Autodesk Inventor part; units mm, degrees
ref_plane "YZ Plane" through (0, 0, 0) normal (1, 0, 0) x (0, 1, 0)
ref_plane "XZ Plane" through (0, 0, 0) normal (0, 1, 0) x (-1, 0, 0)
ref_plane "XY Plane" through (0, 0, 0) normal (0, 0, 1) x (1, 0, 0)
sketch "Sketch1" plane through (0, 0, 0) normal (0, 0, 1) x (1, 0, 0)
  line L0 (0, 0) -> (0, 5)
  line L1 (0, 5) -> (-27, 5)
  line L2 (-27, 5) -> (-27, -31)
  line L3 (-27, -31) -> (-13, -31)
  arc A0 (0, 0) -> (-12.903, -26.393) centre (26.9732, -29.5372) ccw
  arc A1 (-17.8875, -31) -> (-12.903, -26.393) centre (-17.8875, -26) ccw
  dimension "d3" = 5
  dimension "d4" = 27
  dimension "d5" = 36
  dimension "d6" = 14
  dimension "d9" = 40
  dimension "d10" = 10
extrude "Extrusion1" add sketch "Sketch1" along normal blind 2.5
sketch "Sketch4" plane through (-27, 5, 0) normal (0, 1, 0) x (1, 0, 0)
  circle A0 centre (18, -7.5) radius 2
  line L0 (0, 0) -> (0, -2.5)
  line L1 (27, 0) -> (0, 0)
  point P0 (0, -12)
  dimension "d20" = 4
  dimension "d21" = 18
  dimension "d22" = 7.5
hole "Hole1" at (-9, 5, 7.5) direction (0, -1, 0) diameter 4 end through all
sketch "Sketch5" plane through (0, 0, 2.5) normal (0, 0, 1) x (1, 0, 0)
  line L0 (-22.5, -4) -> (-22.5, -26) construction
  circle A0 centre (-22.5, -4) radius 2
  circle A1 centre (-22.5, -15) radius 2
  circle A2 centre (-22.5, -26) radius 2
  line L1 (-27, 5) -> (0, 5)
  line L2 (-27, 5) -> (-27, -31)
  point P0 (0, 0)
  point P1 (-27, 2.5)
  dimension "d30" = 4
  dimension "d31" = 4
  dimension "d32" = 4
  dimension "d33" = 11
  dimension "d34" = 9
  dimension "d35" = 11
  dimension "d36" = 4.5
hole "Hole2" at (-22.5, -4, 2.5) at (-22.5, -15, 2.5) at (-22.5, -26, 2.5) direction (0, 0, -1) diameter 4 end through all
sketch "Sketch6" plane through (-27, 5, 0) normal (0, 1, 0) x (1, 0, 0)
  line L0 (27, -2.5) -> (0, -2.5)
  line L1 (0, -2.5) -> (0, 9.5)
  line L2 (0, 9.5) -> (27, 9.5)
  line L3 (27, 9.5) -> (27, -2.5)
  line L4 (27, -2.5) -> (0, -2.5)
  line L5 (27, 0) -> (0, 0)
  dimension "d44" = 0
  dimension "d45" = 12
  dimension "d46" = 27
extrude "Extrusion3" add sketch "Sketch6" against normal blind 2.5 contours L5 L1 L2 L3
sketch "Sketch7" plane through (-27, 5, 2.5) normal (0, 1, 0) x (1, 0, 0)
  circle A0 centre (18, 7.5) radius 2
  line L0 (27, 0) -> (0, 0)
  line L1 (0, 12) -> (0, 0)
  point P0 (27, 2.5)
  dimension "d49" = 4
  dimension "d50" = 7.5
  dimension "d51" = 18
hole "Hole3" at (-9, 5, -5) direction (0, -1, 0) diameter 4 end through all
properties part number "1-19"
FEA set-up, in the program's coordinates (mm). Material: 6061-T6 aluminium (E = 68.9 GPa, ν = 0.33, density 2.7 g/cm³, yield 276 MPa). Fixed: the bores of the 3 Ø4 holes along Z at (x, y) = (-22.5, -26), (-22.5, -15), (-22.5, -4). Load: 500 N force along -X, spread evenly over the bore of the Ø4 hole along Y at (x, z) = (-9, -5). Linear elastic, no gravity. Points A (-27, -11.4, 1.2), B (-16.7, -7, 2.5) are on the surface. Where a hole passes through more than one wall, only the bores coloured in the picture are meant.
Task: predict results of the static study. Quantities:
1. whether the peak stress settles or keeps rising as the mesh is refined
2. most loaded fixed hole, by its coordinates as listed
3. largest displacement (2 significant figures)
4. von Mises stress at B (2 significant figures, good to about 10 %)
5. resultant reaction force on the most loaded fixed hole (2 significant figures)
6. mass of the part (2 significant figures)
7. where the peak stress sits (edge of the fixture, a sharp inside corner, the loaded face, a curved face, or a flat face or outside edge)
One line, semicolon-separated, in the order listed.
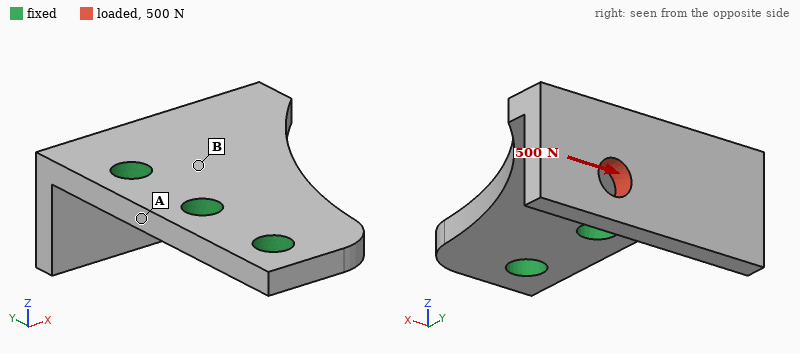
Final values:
keeps rising; (-22.5, -4); 0.20 mm; 66 MPa; 650 N; 6.0 g; edge of the fixture
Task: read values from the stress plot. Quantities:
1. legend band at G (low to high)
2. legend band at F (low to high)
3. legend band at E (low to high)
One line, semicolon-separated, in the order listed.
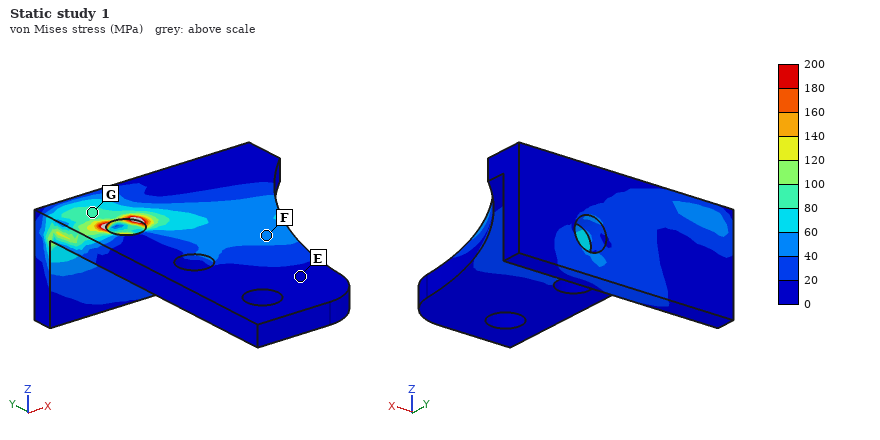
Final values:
80 to 100 MPa; 40 to 60 MPa; 0 to 20 MPa
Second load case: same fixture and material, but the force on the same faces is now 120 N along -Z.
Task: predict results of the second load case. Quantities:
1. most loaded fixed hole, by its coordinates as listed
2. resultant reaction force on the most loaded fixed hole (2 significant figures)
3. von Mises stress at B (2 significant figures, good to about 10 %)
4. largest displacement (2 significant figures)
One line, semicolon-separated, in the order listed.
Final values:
(-22.5, -4); 150 N; 39 MPa; 0.11 mm
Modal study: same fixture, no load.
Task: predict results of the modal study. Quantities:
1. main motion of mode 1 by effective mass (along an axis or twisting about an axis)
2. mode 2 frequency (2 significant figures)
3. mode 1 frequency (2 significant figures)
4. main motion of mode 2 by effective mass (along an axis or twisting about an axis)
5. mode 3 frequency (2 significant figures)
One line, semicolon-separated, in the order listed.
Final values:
along Z; 8300 Hz; 4400 Hz; along Y; 14 kHz
